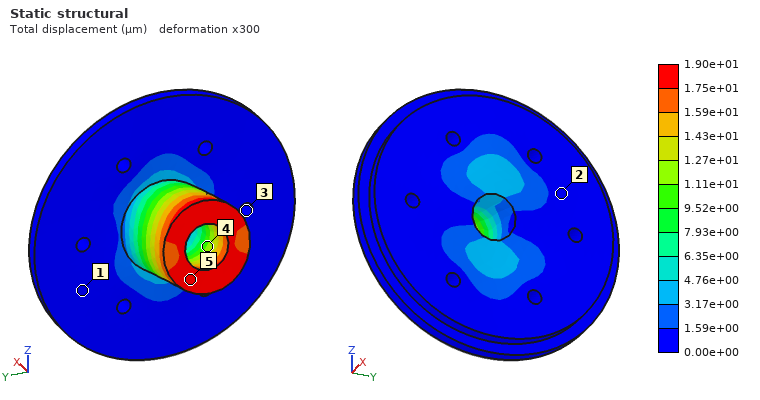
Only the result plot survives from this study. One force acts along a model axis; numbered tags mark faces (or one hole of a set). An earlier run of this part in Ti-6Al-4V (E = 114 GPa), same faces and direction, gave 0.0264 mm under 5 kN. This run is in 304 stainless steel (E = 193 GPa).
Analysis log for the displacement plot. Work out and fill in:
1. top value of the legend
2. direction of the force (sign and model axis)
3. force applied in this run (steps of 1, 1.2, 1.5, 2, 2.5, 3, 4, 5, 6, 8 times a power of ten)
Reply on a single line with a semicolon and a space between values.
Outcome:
1.90e+01 µm; +Z; 6 kN
